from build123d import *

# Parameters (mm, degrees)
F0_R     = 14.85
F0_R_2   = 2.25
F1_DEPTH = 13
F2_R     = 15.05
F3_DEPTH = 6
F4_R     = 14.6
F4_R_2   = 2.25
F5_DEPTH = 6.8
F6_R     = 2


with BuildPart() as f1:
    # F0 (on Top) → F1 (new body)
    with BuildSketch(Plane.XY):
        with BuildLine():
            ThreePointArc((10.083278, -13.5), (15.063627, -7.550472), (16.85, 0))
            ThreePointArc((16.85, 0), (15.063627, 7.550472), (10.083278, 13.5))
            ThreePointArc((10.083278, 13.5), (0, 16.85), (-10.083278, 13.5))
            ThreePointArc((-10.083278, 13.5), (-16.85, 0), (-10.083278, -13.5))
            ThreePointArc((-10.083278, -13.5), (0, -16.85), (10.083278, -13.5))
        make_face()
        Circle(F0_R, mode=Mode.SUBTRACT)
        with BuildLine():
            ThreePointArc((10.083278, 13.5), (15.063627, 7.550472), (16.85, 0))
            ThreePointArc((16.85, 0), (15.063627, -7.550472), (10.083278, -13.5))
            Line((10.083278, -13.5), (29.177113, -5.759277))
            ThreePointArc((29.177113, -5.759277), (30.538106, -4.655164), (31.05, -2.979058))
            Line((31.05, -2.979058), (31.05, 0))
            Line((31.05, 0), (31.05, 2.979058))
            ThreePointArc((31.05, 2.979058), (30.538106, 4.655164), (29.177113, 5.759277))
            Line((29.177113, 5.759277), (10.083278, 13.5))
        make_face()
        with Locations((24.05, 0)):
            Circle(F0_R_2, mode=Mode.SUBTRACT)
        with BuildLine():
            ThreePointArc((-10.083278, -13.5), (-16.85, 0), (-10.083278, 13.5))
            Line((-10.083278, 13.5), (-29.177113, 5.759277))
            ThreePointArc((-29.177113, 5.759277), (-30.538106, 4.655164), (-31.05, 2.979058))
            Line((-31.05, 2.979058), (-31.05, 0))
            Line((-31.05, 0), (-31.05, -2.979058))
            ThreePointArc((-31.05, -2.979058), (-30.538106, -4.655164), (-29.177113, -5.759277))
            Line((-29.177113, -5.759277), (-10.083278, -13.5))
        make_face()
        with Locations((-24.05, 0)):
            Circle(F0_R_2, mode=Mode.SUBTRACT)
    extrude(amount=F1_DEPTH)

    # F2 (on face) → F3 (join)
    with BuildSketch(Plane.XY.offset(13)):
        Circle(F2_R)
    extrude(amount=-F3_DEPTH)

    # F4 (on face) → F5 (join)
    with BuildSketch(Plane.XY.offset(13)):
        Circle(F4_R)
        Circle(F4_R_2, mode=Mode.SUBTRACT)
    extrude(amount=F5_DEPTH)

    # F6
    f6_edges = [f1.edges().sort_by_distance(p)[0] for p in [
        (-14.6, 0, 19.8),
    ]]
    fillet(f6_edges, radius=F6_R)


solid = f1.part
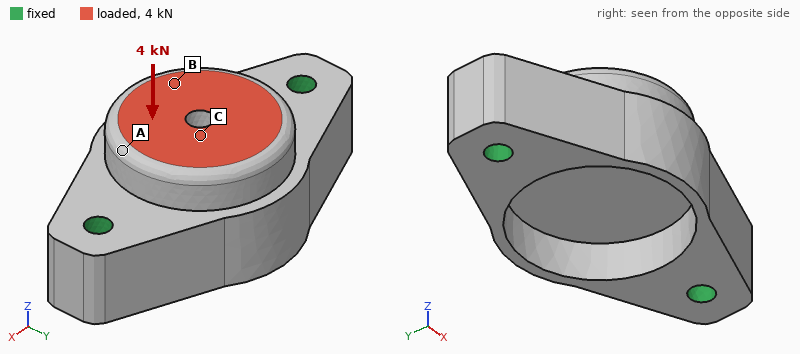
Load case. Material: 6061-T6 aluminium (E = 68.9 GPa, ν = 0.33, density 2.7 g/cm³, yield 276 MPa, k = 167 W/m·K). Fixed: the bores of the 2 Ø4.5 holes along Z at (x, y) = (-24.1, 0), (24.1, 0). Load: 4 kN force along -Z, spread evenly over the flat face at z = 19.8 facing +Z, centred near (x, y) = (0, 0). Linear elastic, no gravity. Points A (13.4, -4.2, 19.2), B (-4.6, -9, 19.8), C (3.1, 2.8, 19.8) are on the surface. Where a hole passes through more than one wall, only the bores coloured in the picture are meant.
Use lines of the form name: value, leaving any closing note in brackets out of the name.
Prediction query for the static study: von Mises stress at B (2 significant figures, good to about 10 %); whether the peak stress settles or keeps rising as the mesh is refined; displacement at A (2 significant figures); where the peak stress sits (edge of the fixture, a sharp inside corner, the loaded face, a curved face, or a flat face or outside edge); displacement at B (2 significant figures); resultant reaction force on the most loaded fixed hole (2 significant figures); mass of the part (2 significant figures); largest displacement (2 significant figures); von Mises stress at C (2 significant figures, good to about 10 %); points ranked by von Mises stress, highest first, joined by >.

von Mises stress at B: 13 MPa
whether the peak stress settles or keeps rising as the mesh is refined: keeps rising
displacement at A: 9.2 µm
where the peak stress sits: edge of the fixture
displacement at B: 13 µm
resultant reaction force on the most loaded fixed hole: 2.4 kN
mass of the part: 47 g
largest displacement: 15 µm
von Mises stress at C: 22 MPa
points ranked by von Mises stress, highest first, joined by >: C > B > A
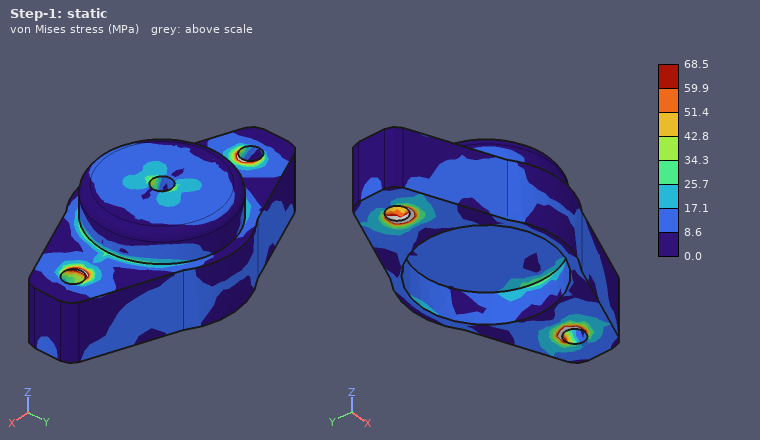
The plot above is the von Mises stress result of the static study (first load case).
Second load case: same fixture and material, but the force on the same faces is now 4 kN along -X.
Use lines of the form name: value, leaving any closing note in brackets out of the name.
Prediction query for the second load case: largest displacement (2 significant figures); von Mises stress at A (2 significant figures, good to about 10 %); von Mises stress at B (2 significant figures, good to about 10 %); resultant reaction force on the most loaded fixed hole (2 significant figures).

largest displacement: 8.1 µm
von Mises stress at A: 6.3 MPa
von Mises stress at B: 15 MPa
resultant reaction force on the most loaded fixed hole: 2.4 kN
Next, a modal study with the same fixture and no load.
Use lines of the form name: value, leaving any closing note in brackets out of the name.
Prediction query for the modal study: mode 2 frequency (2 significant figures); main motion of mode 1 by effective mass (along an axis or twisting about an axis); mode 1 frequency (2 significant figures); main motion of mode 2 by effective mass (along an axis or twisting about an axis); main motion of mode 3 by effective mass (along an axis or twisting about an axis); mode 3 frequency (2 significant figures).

mode 2 frequency: 17 kHz
main motion of mode 1 by effective mass: along Y
mode 1 frequency: 13 kHz
main motion of mode 2 by effective mass: along Z
main motion of mode 3 by effective mass: along Y
mode 3 frequency: 23 kHz
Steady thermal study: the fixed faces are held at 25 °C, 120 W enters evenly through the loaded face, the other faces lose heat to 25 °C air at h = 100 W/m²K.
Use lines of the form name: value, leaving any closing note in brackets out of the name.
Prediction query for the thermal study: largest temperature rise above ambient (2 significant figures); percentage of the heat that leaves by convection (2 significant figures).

largest temperature rise above ambient: 38 K
percentage of the heat that leaves by convection: 7.6 %
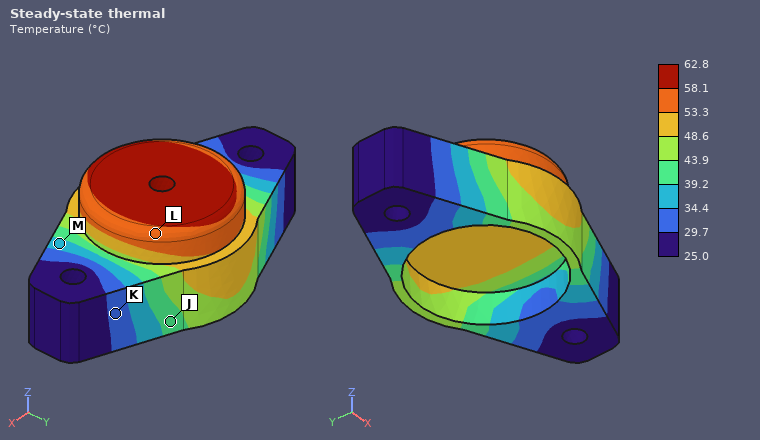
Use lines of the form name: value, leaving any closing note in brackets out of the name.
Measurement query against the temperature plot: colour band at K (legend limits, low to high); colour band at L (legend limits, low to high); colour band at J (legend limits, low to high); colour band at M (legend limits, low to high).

colour band at K: 29.7 to 34.4 °C
colour band at L: 53.3 to 58.1 °C
colour band at J: 39.2 to 43.9 °C
colour band at M: 34.4 to 39.2 °C
